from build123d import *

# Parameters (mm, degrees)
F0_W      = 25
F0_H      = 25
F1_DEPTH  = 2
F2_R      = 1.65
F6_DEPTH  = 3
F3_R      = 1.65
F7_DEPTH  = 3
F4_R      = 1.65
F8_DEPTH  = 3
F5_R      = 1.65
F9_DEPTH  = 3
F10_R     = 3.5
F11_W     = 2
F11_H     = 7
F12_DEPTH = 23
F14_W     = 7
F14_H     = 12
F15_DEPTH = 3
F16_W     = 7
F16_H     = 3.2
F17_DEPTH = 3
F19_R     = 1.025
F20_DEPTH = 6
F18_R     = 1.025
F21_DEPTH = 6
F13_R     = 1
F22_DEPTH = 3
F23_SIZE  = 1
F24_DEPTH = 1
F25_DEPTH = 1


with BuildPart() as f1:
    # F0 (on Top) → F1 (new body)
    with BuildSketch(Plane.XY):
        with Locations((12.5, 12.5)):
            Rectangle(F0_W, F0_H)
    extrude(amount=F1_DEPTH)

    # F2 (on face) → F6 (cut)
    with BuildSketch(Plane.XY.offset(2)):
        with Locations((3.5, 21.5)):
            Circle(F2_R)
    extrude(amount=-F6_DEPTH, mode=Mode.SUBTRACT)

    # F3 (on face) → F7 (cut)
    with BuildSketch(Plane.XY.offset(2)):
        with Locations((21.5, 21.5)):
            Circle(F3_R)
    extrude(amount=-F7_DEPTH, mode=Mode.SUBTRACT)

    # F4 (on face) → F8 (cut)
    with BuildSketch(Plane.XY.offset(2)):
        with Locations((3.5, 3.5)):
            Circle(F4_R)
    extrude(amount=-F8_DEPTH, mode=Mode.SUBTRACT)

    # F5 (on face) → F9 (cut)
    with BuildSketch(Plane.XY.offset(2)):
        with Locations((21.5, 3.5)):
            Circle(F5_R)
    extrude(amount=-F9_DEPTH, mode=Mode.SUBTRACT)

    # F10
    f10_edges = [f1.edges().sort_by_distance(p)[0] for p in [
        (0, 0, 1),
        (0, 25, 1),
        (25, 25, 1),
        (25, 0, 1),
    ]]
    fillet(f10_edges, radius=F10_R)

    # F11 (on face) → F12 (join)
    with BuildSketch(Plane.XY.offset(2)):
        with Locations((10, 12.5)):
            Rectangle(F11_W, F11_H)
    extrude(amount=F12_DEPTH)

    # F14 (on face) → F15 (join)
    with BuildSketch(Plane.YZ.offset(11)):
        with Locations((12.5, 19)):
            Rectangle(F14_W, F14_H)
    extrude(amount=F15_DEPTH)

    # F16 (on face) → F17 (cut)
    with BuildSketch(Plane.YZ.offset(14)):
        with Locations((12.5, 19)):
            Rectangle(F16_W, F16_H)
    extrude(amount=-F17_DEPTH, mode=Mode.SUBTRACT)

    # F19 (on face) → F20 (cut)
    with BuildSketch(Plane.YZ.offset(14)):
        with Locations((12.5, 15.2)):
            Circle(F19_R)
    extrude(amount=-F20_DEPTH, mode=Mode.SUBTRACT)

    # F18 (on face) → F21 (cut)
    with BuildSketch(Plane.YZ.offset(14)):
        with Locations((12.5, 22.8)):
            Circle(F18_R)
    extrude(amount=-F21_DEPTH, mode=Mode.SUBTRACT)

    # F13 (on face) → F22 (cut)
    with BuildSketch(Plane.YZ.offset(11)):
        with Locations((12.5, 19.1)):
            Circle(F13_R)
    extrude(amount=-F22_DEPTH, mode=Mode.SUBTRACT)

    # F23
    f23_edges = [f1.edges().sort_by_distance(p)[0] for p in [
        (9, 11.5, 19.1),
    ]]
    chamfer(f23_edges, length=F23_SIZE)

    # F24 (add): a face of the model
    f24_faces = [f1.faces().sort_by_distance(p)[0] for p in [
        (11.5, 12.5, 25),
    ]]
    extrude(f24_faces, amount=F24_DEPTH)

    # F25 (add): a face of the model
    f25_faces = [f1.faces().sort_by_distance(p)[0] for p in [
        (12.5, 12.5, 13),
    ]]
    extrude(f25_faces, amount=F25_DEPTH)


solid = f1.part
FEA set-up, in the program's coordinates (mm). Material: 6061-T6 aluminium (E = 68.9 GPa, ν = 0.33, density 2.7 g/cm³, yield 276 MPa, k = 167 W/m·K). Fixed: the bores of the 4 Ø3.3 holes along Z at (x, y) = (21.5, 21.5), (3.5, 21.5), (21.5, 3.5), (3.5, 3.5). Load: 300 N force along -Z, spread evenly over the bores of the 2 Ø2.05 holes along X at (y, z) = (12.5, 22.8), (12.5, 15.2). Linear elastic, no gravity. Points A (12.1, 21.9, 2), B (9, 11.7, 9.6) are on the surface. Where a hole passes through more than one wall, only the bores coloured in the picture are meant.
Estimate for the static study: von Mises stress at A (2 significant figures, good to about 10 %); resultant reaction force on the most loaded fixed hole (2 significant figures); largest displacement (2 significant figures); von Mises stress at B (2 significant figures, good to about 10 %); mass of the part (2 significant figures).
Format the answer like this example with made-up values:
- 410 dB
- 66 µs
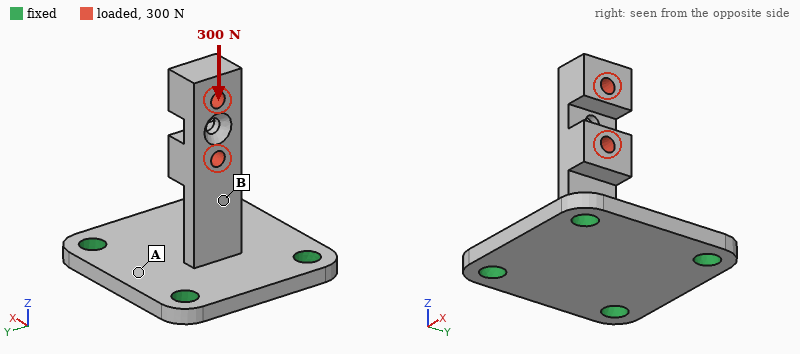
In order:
- 19 MPa
- 88 N
- 0.37 mm
- 67 MPa
- 4.5 g
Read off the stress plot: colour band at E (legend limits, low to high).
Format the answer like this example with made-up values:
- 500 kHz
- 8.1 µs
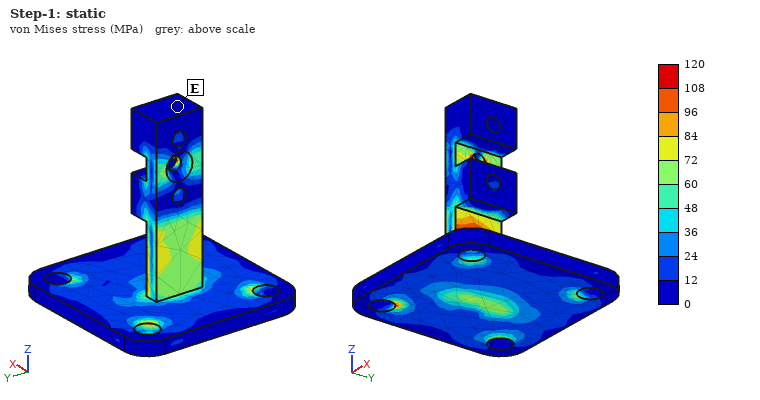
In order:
- 0 to 12 MPa
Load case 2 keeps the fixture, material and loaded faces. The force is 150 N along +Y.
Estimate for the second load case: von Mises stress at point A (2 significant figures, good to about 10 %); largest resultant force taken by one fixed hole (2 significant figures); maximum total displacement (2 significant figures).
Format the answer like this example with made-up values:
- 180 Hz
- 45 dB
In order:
- 22 MPa
- 150 N
- 0.22 mm
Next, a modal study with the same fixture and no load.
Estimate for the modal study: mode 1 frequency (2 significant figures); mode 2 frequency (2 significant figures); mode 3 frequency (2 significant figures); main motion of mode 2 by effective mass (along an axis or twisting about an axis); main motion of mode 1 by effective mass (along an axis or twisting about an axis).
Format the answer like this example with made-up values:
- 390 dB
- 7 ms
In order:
- 1900 Hz
- 4800 Hz
- 12 kHz
- along Y
- along X
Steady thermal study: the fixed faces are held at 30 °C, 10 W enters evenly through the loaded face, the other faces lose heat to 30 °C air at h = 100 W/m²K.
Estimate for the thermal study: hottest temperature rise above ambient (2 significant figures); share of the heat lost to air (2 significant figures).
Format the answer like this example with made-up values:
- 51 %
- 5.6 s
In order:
- 62 K
- 29 %
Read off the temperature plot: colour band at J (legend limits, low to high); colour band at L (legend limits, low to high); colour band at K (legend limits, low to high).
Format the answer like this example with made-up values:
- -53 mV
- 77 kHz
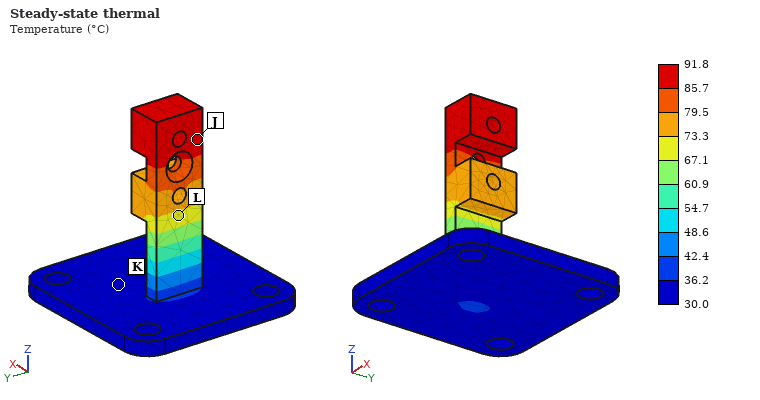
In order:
- 85.7 to 91.8 °C
- 67.1 to 73.3 °C
- 30.0 to 36.2 °C
